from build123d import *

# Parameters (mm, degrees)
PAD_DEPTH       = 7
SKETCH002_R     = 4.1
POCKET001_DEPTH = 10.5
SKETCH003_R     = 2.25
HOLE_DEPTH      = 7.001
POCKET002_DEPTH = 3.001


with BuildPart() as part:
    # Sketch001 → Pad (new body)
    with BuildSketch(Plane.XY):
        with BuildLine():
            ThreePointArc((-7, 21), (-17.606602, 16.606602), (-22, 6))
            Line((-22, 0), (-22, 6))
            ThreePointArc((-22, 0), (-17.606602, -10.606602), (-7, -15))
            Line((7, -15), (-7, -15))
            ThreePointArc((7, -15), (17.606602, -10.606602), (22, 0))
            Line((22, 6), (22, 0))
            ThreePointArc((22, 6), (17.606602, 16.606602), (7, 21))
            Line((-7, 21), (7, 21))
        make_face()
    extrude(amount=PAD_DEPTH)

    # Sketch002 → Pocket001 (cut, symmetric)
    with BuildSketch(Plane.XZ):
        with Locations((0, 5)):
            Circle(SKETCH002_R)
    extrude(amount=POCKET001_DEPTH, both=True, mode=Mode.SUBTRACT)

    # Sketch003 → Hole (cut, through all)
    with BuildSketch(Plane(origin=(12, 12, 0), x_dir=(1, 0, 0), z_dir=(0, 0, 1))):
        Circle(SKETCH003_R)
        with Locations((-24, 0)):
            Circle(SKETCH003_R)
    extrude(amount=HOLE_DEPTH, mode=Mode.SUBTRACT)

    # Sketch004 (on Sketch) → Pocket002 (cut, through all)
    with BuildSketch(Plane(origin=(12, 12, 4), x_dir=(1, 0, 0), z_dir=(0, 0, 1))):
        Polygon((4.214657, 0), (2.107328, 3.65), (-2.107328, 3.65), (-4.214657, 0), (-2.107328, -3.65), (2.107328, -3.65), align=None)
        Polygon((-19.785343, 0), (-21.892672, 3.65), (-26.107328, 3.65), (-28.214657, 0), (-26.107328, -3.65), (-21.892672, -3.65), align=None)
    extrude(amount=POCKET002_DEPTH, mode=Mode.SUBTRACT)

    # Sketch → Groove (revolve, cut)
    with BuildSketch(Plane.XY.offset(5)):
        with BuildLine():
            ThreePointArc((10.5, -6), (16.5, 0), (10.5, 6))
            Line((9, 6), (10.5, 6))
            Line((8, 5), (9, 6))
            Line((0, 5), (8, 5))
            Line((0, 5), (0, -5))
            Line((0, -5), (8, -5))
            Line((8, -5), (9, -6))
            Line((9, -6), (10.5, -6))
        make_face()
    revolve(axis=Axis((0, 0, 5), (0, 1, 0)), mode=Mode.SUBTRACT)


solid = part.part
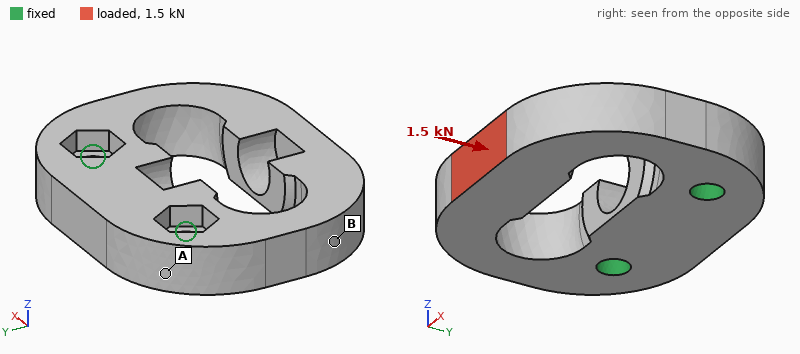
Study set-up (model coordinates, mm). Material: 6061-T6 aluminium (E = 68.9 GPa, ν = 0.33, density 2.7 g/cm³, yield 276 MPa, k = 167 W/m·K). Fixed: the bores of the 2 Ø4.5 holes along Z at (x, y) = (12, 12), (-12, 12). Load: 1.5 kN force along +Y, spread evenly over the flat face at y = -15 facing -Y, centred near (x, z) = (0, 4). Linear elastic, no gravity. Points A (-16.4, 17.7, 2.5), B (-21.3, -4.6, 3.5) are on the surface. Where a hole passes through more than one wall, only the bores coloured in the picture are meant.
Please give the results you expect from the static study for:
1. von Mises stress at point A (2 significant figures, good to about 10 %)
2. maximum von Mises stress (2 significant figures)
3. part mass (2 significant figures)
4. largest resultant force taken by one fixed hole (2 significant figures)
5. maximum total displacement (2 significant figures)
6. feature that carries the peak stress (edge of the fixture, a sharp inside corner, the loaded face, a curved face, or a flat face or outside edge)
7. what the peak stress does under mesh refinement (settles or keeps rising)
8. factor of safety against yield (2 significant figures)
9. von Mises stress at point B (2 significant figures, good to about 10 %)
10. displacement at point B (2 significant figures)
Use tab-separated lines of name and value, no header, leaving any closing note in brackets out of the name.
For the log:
von Mises stress at point A	22 MPa
maximum von Mises stress	320 MPa
part mass	18 g
largest resultant force taken by one fixed hole	910 N
maximum total displacement	62 µm
feature that carries the peak stress	a curved face
what the peak stress does under mesh refinement	settles
factor of safety against yield	0.86
von Mises stress at point B	44 MPa
displacement at point B	17 µm
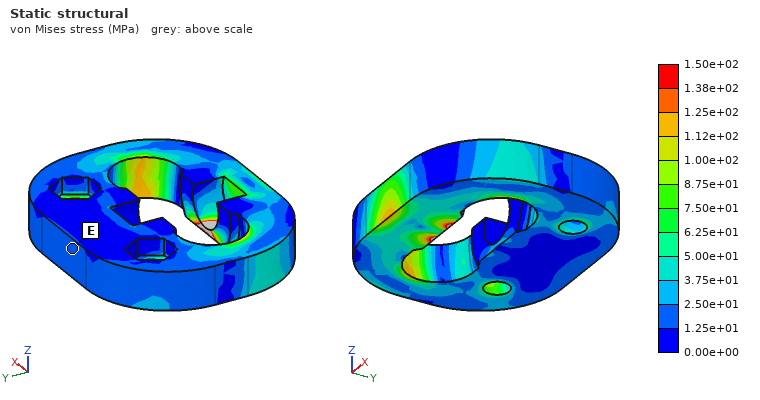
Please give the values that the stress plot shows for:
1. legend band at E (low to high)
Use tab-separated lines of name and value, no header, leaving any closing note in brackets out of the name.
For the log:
legend band at E	1.25e+01 to 2.50e+01 MPa
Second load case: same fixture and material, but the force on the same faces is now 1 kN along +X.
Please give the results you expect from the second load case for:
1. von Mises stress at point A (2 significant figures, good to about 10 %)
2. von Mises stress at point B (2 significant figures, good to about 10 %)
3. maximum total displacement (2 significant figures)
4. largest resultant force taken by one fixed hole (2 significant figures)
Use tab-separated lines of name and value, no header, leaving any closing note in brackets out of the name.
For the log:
von Mises stress at point A	25 MPa
von Mises stress at point B	18 MPa
maximum total displacement	47 µm
largest resultant force taken by one fixed hole	940 N
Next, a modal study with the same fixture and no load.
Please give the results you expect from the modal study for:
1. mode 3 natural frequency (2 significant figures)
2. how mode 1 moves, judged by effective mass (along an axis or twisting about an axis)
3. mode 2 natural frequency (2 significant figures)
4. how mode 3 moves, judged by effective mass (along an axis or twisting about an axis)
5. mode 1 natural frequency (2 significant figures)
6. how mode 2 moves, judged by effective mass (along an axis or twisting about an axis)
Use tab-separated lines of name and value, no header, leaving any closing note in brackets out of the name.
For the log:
mode 3 natural frequency	9700 Hz
how mode 1 moves, judged by effective mass	along Z
mode 2 natural frequency	9300 Hz
how mode 3 moves, judged by effective mass	along X
mode 1 natural frequency	4300 Hz
how mode 2 moves, judged by effective mass	along X
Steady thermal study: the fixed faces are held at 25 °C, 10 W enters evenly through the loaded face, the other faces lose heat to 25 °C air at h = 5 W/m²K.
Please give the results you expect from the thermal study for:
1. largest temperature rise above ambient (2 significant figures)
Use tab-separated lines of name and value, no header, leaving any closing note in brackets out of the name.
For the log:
largest temperature rise above ambient	22 K
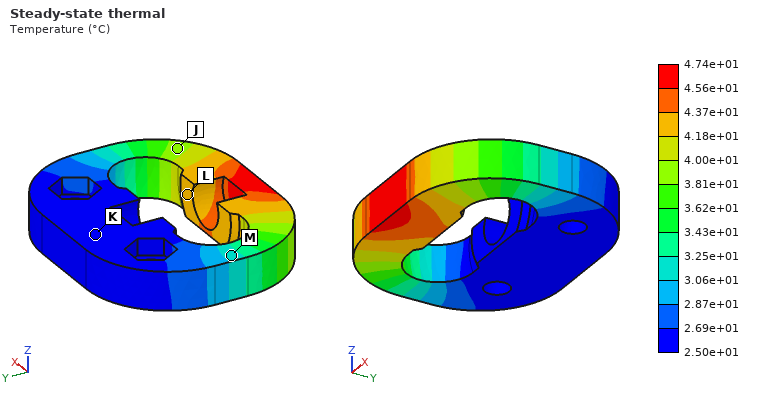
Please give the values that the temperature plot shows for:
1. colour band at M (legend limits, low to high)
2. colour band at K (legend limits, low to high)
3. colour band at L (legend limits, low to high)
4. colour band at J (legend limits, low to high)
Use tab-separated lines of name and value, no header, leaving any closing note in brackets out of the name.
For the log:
colour band at M	3.06e+01 to 3.25e+01 °C
colour band at K	2.50e+01 to 2.69e+01 °C
colour band at L	4.18e+01 to 4.37e+01 °C
colour band at J	3.81e+01 to 4.00e+01 °C
